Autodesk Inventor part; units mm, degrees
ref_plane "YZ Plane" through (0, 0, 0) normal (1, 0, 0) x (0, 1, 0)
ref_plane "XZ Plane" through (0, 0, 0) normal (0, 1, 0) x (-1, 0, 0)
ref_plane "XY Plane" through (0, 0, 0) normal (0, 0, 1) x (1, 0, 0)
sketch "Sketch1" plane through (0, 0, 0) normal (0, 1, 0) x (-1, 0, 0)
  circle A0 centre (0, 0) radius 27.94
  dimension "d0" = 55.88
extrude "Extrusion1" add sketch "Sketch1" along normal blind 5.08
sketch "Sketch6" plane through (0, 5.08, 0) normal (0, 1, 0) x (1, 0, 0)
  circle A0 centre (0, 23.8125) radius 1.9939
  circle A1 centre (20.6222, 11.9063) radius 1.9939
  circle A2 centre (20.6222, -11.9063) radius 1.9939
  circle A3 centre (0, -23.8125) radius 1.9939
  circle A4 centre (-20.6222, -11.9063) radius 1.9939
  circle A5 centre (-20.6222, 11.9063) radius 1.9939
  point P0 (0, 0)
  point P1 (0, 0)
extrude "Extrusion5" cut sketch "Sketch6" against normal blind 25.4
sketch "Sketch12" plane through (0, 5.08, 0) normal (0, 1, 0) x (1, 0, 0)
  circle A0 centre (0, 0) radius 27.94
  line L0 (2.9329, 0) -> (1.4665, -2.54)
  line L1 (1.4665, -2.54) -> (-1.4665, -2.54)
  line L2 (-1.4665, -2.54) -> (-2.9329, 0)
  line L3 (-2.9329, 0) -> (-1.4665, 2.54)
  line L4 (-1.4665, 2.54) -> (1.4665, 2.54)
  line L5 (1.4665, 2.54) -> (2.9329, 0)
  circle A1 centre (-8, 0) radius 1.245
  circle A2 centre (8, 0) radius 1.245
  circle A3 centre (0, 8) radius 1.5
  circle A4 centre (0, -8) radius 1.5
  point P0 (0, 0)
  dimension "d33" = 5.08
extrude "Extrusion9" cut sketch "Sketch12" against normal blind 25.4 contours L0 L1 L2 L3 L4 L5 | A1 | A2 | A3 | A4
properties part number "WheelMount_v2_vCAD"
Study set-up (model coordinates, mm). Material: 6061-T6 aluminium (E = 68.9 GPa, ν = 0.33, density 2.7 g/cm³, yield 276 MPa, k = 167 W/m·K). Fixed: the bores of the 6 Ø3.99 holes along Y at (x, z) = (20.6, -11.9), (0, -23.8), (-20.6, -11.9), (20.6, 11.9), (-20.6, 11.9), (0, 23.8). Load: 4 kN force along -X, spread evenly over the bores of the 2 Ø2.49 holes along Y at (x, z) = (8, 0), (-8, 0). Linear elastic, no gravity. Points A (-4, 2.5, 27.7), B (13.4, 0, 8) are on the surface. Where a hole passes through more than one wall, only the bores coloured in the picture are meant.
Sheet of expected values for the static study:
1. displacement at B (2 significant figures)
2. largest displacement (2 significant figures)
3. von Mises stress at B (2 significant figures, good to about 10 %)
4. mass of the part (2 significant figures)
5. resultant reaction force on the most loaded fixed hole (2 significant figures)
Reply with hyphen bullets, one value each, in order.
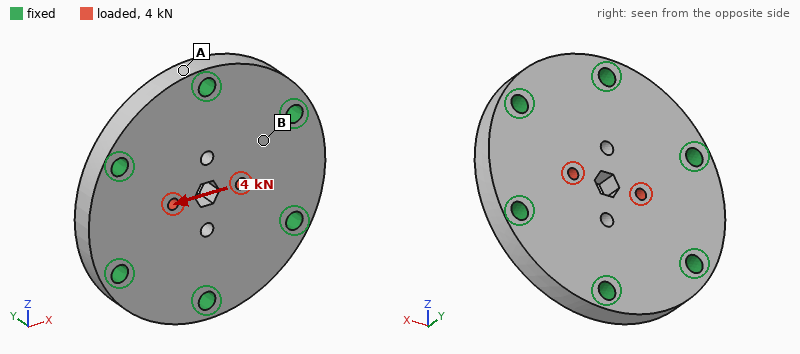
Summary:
- 2.0 µm
- 7.1 µm
- 18 MPa
- 32 g
- 930 N
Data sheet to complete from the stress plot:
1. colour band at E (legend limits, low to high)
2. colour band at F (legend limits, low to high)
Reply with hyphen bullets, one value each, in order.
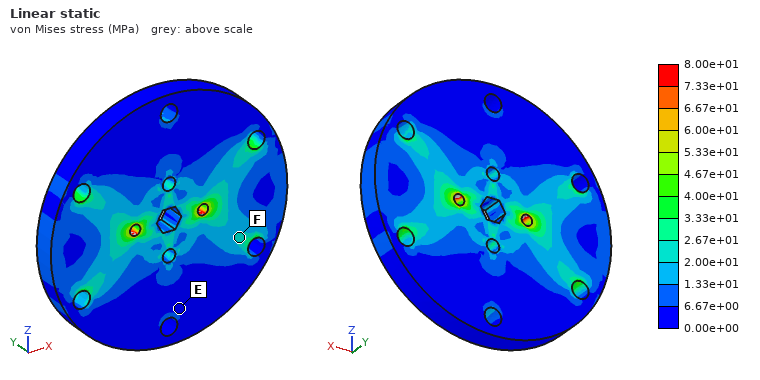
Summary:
- 0.00e+00 to 6.67e+00 MPa
- 2.00e+01 to 2.67e+01 MPa
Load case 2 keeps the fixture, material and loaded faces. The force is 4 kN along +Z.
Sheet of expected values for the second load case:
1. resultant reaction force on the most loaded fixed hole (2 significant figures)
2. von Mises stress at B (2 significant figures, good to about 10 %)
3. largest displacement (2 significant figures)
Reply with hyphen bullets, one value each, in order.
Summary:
- 860 N
- 13 MPa
- 5.7 µm
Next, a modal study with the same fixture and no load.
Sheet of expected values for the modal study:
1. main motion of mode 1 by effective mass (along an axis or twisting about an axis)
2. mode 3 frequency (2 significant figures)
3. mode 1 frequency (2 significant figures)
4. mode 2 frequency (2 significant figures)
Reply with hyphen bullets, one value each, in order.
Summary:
- along Y
- 33 kHz
- 18 kHz
- 33 kHz
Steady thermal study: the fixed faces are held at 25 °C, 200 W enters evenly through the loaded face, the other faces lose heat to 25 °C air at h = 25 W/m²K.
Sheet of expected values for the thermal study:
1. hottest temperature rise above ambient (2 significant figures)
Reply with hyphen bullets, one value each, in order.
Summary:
- 71 K
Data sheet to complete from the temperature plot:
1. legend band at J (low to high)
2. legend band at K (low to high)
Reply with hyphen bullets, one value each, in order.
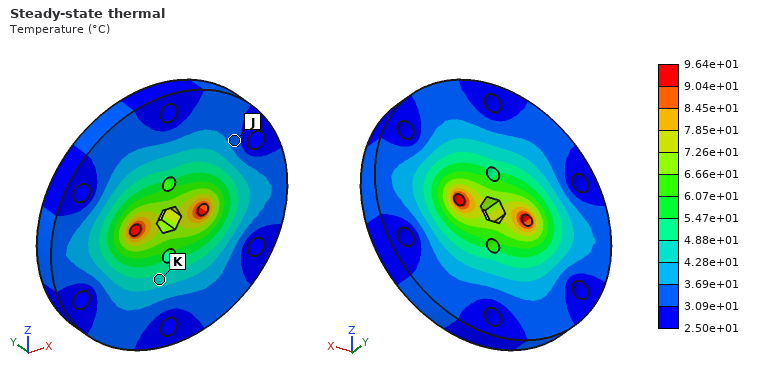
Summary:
- 3.09e+01 to 3.69e+01 °C
- 4.28e+01 to 4.88e+01 °C
